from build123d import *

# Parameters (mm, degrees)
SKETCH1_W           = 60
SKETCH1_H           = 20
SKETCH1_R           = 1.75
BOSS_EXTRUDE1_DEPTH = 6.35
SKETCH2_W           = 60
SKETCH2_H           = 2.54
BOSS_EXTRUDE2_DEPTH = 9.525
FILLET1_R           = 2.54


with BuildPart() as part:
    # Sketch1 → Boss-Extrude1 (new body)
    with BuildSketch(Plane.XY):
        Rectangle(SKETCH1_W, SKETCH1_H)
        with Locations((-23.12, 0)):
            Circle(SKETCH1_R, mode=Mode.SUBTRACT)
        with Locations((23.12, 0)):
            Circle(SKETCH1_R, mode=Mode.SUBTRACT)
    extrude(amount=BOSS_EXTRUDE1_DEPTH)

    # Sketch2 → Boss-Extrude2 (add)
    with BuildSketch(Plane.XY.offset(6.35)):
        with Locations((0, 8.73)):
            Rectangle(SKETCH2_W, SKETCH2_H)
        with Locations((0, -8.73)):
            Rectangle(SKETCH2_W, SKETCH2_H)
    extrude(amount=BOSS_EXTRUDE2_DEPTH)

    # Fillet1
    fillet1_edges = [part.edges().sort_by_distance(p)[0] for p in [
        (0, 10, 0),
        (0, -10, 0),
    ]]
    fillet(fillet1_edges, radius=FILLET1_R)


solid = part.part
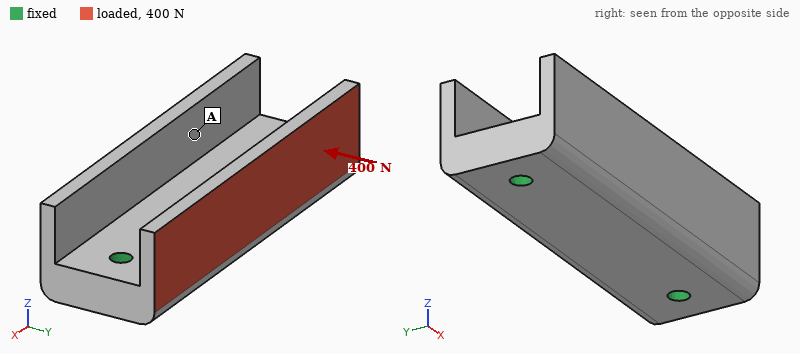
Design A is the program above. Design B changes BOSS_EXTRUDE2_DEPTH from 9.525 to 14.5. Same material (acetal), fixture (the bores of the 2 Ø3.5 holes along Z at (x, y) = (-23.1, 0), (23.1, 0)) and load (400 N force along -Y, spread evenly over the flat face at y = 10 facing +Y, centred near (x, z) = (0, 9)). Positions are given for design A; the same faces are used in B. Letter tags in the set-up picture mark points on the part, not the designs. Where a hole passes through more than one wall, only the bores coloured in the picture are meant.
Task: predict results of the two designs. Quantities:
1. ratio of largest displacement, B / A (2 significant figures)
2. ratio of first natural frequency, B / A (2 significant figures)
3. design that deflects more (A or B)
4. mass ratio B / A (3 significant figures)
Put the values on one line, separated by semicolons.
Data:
2.5; 0.64; B; 1.15
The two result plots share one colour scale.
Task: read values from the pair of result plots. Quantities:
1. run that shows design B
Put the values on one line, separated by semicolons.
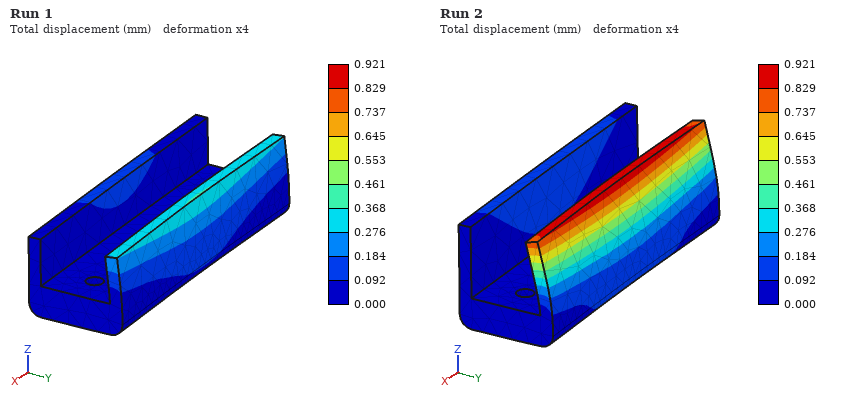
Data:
Run 2
